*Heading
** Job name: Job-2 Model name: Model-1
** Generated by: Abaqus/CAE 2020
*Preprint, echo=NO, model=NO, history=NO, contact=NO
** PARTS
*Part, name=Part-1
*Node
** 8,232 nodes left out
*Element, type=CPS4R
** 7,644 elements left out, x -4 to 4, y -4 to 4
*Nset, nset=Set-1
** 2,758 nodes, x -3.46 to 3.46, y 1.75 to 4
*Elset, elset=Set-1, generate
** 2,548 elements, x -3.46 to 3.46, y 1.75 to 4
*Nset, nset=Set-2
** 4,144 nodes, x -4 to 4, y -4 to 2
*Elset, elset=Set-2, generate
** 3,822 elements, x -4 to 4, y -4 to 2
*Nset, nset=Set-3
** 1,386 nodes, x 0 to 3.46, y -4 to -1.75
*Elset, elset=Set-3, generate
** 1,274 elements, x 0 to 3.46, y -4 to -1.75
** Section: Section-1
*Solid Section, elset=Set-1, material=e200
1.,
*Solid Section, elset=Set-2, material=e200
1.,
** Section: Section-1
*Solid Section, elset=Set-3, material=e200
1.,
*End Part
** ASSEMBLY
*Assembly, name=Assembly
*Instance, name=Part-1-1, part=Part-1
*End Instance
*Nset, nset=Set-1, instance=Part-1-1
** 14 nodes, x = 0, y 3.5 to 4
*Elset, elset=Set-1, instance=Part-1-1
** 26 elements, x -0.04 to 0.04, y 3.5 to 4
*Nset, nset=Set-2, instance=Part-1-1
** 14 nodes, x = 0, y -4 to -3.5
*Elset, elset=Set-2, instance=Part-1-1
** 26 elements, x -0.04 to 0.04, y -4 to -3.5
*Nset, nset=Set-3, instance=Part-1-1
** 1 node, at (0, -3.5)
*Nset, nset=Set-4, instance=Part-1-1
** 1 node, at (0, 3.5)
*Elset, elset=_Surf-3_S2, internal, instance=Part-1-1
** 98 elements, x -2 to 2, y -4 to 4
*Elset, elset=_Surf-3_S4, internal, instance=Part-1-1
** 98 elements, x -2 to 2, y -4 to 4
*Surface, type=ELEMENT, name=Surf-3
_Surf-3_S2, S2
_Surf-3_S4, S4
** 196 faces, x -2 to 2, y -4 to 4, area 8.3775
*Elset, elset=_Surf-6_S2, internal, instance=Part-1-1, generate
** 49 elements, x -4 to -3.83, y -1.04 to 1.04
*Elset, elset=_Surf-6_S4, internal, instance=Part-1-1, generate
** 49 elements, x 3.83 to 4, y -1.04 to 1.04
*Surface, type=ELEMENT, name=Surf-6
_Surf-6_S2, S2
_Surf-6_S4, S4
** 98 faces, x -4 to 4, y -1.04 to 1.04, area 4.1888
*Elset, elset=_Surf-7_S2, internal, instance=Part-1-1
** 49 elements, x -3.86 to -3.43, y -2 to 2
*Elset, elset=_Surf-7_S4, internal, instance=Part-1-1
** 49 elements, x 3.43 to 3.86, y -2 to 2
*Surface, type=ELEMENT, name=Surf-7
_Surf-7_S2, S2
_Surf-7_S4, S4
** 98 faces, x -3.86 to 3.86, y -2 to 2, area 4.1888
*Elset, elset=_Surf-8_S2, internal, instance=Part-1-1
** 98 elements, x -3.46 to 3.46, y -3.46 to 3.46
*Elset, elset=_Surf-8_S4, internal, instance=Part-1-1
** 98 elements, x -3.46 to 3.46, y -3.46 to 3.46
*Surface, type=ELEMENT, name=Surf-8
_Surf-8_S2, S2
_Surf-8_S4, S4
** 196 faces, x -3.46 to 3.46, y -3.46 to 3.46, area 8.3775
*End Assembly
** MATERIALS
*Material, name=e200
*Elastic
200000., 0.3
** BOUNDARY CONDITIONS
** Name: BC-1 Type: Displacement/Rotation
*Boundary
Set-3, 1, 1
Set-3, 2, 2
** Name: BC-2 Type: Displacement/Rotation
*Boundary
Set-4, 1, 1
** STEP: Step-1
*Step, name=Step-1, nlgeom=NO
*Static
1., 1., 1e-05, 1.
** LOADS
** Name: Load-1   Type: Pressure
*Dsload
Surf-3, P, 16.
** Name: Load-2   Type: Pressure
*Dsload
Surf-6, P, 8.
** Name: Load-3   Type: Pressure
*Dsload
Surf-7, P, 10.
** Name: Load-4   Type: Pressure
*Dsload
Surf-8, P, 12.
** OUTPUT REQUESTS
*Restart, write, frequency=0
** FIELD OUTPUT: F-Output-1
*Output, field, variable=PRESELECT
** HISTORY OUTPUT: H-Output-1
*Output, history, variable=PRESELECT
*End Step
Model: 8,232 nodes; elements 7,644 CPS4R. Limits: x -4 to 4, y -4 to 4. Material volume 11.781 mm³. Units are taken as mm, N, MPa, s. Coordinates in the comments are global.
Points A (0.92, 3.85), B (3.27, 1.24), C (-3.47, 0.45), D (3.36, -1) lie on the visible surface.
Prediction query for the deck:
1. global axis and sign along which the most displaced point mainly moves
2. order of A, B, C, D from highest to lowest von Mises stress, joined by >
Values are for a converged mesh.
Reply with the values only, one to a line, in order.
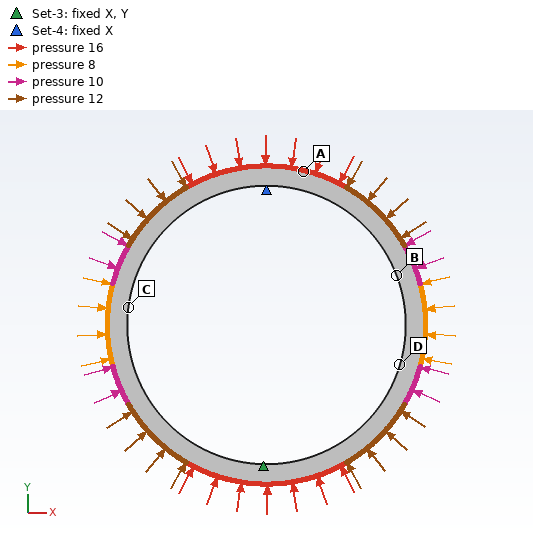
-Y
C > D > B > A
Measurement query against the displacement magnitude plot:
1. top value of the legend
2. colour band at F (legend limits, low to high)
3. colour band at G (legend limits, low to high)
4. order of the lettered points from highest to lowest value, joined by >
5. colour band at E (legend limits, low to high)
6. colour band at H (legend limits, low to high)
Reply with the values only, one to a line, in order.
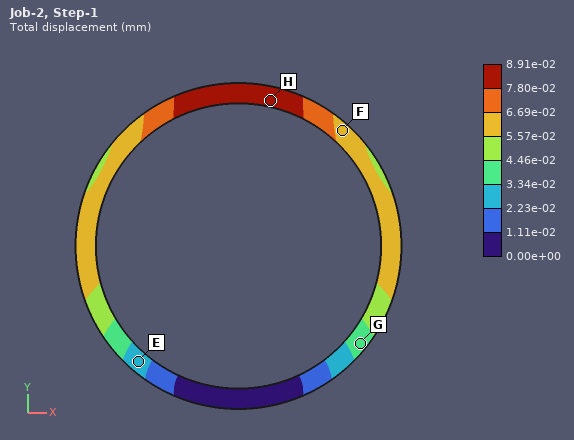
8.91e-02 mm
5.57e-02 to 6.69e-02 mm
3.34e-02 to 4.46e-02 mm
H > F > G > E
2.23e-02 to 3.34e-02 mm
7.80e-02 to 8.91e-02 mm
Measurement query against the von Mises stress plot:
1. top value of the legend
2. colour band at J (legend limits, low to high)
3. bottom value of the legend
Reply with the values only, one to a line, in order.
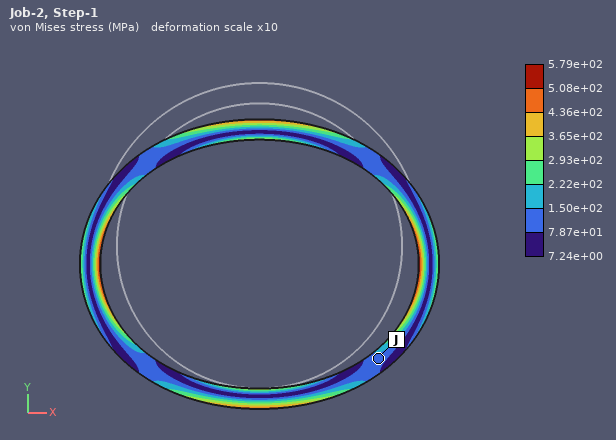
5.79e+02 MPa
7.87e+01 to 1.50e+02 MPa
7.24e+00 MPa
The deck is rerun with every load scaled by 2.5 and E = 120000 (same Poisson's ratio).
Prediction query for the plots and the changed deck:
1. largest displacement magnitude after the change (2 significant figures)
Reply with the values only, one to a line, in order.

0.37 mm
